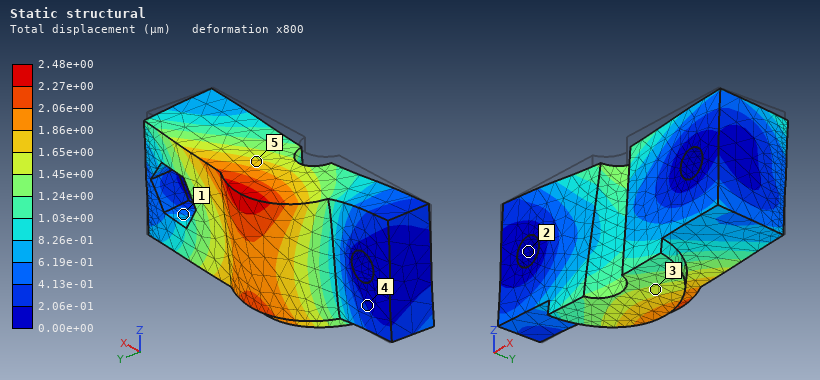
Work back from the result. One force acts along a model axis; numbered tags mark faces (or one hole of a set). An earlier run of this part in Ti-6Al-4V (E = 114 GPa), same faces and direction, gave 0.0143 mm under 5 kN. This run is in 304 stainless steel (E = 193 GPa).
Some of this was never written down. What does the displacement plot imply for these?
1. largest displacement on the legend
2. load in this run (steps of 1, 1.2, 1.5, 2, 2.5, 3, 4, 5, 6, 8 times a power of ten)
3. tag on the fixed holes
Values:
2.48e+00 µm
1.5 kN
2
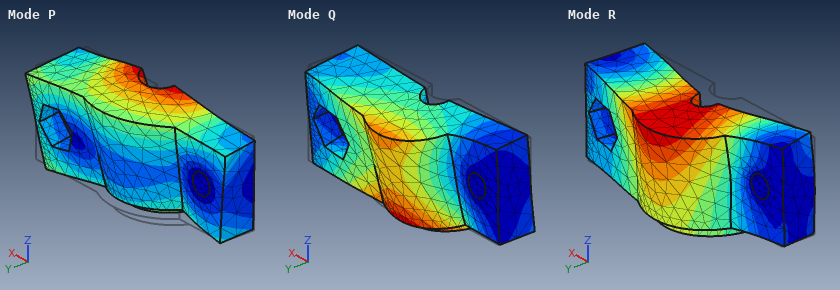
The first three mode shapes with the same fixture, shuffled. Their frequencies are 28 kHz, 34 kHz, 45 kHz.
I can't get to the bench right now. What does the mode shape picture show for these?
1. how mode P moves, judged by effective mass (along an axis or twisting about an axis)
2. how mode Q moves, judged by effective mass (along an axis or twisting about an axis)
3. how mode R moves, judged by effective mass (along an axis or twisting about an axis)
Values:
along Z
along Z
along Y
